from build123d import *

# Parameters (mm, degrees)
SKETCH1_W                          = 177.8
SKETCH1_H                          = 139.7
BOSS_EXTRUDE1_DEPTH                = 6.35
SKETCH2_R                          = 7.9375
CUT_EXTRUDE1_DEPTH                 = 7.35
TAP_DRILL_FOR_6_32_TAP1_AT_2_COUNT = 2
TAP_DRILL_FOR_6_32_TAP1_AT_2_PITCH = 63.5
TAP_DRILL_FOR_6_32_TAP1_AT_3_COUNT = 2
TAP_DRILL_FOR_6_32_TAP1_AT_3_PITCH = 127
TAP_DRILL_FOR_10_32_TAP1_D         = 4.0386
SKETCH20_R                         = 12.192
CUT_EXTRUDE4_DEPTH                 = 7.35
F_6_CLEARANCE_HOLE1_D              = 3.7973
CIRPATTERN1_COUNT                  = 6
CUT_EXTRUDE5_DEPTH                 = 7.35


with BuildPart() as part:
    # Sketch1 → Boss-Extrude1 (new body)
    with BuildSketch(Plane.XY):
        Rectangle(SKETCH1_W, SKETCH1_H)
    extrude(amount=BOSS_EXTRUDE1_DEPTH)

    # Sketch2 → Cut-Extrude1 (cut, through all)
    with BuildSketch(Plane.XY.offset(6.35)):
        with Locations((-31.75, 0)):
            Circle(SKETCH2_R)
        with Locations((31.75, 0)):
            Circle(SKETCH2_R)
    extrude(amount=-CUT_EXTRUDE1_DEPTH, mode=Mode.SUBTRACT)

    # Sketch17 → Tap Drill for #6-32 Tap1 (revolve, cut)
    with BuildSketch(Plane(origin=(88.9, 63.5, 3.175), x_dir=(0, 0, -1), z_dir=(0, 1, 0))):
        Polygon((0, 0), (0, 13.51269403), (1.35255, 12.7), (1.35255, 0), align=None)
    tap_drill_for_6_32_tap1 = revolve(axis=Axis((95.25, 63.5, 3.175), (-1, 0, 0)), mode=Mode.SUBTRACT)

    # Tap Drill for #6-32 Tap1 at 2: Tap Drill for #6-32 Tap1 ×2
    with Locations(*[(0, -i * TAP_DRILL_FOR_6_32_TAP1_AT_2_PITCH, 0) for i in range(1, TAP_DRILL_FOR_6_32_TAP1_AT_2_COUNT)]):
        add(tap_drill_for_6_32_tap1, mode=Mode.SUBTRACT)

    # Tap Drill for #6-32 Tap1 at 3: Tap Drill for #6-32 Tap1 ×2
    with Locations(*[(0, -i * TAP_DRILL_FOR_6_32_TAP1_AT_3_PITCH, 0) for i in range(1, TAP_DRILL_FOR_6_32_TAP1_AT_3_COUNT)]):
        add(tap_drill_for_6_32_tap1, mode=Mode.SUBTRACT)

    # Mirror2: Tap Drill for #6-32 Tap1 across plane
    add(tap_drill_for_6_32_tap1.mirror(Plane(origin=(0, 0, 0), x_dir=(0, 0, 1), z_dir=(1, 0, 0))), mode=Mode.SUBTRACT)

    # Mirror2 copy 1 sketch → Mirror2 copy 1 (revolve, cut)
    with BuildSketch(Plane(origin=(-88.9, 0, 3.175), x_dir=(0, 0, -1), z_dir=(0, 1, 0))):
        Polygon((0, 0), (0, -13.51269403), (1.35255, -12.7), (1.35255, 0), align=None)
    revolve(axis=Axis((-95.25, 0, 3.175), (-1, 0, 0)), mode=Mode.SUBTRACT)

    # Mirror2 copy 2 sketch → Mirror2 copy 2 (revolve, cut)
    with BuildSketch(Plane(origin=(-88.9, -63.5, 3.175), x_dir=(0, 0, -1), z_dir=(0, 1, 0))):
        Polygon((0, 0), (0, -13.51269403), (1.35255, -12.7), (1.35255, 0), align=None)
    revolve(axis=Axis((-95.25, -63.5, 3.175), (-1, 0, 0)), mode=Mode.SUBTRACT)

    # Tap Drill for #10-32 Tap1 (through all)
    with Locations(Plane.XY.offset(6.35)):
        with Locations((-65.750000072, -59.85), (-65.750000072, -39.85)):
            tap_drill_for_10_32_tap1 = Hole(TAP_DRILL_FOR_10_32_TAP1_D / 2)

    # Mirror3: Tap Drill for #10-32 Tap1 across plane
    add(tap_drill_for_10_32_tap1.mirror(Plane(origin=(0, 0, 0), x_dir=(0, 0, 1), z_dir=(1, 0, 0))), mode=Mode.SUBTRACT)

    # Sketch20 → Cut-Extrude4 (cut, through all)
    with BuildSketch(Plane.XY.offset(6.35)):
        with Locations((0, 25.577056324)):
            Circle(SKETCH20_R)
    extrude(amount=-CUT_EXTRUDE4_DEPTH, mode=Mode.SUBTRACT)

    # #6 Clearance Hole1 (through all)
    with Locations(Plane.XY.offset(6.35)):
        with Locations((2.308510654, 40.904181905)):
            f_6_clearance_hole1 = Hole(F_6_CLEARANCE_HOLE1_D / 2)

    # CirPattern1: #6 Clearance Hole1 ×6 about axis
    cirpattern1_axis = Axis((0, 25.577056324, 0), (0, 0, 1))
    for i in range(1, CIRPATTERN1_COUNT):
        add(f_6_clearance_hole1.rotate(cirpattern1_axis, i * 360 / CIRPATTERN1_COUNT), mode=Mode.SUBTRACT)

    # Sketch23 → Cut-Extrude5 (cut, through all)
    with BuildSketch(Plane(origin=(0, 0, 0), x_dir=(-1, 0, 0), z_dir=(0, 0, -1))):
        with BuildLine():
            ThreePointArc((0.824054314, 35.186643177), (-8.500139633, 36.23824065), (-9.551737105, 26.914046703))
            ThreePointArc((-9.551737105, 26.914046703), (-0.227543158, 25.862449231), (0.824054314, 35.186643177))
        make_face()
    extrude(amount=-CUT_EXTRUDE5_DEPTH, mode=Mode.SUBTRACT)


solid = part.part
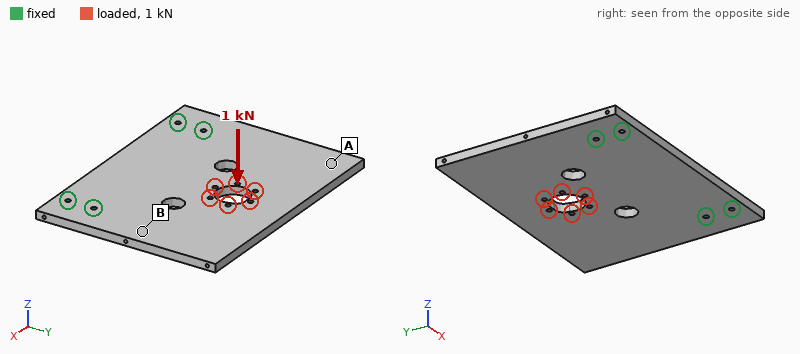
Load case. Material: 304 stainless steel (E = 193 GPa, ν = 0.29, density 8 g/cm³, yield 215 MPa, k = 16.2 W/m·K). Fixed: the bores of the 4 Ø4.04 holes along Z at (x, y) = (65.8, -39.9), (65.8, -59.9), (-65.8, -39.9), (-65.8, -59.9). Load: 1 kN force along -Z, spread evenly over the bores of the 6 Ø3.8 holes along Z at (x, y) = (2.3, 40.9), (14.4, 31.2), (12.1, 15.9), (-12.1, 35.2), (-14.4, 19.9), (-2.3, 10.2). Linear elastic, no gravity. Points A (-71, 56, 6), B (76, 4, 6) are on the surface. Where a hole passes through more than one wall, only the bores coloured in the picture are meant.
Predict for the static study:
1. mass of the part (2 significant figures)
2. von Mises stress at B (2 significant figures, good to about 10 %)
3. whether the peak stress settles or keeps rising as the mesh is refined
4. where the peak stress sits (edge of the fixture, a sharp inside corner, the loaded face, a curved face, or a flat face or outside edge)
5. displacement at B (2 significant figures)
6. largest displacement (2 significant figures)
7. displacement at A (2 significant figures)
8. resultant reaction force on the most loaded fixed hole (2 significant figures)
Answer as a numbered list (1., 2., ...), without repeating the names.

1. 1.2 kg
2. 27 MPa
3. keeps rising
4. edge of the fixture
5. 0.092 mm
6. 0.47 mm
7. 0.31 mm
8. 1.4 kN
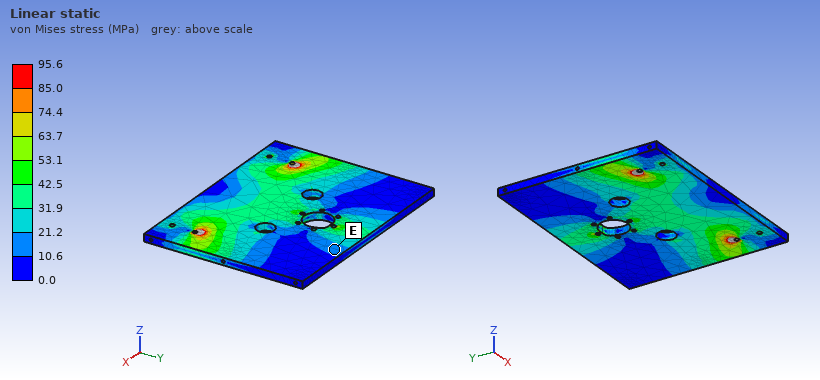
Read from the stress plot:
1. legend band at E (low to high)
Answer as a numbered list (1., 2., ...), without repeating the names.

1. 10.6 to 21.2 MPa
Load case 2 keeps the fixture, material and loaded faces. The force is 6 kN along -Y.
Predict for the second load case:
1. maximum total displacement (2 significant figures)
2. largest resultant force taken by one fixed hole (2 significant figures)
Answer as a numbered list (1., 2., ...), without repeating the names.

1. 8.3 µm
2. 2.0 kN
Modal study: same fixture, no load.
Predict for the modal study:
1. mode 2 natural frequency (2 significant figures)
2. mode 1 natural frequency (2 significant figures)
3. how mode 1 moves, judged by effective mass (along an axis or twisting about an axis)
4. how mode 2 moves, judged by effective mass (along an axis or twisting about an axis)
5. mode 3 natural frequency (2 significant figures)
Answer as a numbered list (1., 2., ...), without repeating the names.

1. 690 Hz
2. 350 Hz
3. along Z
4. twisting about Y
5. 1300 Hz
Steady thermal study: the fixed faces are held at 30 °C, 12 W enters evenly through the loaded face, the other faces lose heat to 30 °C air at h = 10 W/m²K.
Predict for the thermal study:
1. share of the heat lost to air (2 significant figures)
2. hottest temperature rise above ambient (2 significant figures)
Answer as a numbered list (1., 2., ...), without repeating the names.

1. 69 %
2. 48 K
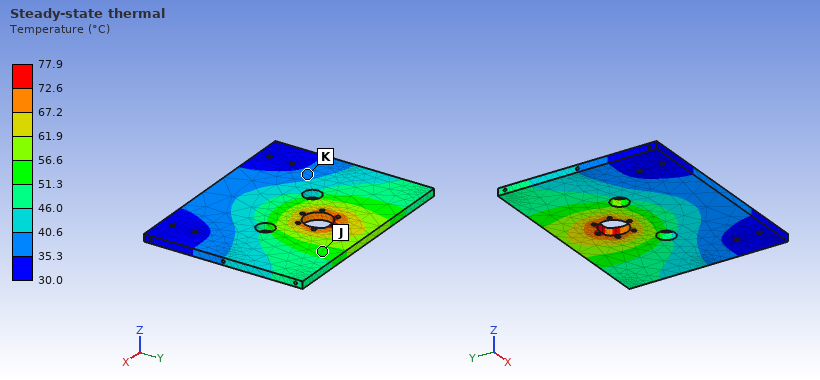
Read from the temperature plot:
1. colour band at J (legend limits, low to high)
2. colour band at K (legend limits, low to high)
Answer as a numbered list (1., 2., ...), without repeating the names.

1. 51.3 to 56.6 °C
2. 35.3 to 40.6 °C
